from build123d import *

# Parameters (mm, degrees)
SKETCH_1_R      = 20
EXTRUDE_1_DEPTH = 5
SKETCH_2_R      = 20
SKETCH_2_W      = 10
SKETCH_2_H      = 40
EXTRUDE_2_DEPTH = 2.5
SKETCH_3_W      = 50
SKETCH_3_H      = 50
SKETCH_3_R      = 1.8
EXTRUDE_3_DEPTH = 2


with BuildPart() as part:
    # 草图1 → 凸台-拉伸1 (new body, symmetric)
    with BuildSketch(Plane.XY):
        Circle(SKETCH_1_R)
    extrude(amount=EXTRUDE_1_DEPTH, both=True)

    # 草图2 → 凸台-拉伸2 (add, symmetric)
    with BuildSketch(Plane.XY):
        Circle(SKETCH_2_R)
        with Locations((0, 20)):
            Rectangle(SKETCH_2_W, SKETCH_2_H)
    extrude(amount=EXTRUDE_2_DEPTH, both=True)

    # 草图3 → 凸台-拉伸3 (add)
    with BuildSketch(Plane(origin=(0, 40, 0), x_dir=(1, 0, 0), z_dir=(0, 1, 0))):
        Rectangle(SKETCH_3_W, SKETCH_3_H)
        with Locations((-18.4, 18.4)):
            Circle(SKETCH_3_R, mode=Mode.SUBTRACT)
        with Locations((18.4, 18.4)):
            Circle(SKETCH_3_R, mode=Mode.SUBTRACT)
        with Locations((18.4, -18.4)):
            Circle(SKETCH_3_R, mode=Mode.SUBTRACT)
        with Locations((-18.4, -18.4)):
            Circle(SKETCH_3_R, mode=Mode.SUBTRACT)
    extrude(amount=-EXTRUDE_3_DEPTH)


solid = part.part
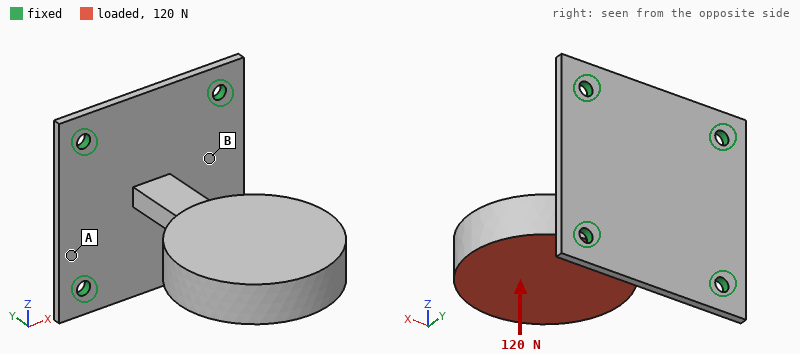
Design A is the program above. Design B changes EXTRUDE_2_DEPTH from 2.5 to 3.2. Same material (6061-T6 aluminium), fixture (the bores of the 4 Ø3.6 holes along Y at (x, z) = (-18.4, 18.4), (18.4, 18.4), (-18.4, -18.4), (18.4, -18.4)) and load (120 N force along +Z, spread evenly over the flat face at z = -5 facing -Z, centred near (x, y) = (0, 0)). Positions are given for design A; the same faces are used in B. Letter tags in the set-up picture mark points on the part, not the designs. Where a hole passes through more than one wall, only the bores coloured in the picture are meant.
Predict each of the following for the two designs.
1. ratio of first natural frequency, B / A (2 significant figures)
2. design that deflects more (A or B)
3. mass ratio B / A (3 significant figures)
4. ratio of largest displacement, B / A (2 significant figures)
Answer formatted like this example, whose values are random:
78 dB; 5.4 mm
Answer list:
1.2; A; 1.01; 0.69
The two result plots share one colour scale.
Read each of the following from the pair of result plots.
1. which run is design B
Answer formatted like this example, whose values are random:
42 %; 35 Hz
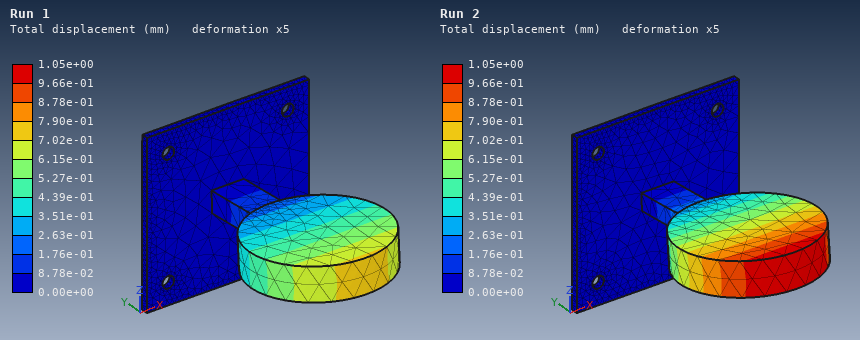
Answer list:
Run 1
